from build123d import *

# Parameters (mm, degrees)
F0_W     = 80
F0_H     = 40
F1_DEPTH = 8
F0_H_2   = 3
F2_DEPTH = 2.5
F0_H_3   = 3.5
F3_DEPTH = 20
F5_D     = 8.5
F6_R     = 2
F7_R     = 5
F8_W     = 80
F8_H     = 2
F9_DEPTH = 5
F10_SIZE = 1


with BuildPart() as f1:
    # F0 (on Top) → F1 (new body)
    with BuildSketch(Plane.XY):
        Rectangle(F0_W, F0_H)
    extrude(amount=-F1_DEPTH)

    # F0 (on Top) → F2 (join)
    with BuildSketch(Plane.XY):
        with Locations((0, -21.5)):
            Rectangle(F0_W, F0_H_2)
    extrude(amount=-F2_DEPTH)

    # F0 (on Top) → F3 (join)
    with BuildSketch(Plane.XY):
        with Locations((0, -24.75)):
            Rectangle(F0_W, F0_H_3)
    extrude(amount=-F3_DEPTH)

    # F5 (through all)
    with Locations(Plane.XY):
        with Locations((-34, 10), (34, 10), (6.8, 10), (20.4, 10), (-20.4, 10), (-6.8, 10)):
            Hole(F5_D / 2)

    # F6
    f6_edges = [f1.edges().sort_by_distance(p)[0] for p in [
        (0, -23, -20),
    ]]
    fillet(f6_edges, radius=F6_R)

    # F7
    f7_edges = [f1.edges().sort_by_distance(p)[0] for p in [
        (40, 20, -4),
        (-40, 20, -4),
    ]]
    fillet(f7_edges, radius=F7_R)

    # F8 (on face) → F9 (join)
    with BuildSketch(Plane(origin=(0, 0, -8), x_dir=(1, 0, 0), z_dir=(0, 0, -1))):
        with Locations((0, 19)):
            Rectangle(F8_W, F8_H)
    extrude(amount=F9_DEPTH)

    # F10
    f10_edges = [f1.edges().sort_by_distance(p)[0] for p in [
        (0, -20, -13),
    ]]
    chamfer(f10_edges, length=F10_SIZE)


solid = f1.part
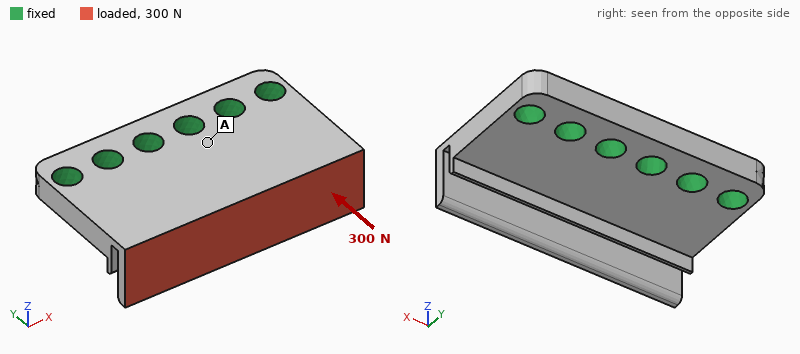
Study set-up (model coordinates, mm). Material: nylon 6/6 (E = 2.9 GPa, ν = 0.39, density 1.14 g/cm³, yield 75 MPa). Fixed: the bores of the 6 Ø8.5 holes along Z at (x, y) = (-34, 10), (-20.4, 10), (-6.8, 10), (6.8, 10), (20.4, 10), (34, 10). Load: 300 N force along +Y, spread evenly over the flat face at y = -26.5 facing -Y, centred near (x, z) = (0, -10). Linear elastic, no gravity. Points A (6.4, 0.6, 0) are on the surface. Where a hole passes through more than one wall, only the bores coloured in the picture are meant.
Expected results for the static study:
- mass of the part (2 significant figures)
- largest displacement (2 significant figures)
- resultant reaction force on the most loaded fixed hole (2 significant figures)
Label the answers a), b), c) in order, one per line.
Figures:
a) 34 g
b) 0.96 mm
c) 58 N
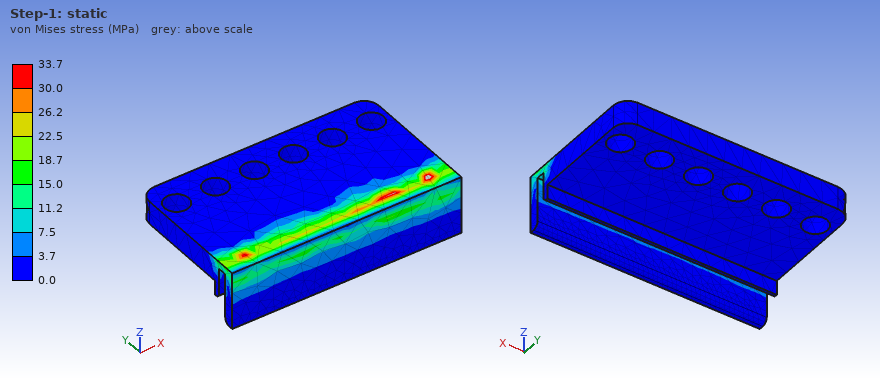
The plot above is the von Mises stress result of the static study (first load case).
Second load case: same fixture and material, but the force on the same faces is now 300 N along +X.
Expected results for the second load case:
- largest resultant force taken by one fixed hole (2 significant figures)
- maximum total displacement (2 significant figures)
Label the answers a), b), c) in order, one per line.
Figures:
a) 130 N
b) 0.16 mm
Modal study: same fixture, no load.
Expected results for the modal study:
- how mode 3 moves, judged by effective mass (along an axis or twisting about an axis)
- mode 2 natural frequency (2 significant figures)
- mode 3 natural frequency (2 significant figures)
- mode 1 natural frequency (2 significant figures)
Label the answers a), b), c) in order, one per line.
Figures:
a) along Z
b) 1600 Hz
c) 1900 Hz
d) 1200 Hz
